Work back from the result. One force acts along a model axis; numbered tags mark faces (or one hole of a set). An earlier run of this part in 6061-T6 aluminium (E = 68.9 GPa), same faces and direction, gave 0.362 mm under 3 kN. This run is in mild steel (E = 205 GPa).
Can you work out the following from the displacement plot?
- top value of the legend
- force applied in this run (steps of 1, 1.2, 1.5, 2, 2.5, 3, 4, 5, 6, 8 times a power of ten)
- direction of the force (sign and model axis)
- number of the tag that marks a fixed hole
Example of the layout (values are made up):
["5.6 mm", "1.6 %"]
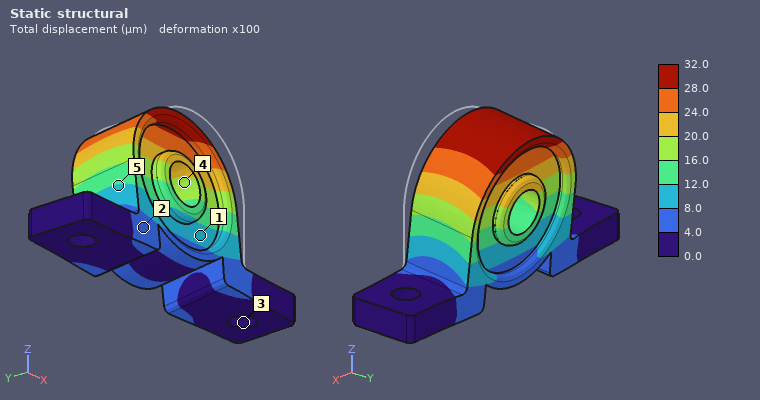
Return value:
["32.0 µm", "800 N", "+Y", "3"]
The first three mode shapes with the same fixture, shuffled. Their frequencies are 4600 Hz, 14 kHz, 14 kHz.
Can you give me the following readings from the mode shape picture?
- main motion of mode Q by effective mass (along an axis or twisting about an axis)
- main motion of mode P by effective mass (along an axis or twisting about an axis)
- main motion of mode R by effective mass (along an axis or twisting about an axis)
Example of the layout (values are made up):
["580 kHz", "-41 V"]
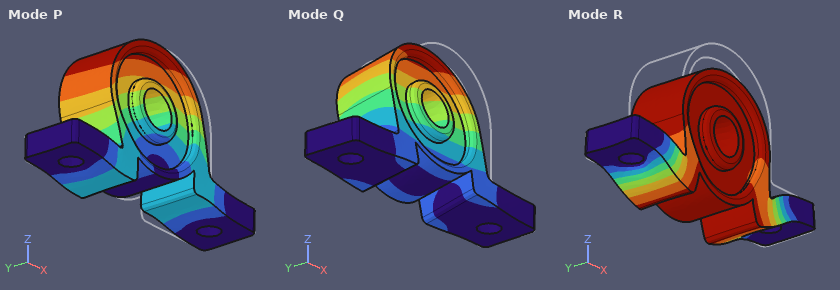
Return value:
["along Y", "along X", "along Z"]
